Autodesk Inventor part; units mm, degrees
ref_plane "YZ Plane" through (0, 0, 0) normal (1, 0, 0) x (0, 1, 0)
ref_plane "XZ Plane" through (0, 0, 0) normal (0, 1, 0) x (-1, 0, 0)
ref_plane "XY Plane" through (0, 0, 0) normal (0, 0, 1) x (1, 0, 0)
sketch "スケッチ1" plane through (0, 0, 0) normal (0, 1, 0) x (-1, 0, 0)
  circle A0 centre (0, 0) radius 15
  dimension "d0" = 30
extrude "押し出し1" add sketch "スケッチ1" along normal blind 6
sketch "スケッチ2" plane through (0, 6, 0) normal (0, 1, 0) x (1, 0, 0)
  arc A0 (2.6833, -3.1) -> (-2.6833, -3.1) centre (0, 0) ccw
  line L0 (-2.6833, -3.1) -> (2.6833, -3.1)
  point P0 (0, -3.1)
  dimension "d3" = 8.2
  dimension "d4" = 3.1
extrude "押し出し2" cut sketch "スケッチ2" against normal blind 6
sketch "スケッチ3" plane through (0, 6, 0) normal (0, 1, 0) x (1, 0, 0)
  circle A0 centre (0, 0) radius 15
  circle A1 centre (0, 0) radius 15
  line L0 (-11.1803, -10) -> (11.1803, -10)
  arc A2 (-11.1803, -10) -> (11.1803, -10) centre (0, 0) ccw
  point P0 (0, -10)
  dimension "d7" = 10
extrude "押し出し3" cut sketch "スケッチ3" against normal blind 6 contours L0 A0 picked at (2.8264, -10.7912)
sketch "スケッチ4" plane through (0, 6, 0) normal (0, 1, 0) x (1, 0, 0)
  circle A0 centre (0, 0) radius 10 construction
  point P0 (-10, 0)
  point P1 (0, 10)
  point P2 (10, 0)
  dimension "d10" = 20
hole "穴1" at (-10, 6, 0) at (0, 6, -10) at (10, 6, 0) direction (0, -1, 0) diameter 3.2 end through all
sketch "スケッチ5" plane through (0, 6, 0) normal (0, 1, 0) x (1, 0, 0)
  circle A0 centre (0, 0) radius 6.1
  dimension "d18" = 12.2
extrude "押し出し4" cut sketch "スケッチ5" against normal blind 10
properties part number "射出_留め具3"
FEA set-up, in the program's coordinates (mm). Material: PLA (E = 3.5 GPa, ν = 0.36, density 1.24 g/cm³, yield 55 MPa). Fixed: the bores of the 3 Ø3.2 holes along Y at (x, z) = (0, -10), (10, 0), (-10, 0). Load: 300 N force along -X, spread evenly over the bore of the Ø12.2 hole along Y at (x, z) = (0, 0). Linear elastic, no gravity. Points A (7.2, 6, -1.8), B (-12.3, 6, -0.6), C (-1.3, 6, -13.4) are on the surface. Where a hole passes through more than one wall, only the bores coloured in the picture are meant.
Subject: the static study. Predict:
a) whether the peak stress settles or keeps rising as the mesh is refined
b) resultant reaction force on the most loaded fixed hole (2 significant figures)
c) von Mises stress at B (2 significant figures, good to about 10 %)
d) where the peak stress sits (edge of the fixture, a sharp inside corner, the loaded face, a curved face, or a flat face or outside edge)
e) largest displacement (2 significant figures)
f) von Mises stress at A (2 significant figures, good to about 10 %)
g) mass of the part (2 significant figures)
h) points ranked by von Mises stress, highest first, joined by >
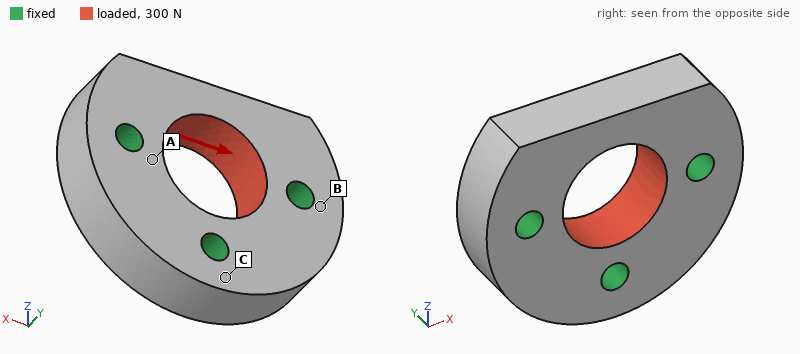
keeps rising
120 N
1.0 MPa
edge of the fixture
12 µm
2.2 MPa
3.6 g
A > B > C
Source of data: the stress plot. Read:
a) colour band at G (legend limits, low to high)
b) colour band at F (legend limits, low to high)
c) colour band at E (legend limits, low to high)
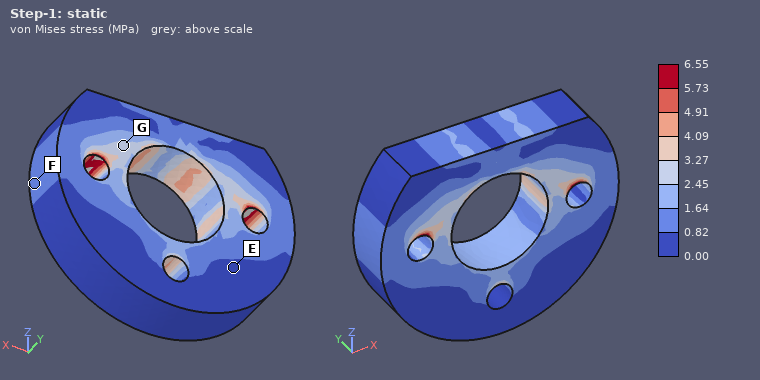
2.45 to 3.27 MPa
0.82 to 1.64 MPa
0.00 to 0.82 MPa
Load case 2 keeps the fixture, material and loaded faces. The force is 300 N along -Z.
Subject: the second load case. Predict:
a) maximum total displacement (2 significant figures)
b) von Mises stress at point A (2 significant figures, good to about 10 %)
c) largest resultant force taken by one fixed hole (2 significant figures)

14 µm
1.9 MPa
110 N
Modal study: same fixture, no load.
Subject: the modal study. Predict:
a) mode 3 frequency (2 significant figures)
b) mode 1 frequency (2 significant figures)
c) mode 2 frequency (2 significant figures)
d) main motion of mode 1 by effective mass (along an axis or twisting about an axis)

17 kHz
11 kHz
16 kHz
along Y
